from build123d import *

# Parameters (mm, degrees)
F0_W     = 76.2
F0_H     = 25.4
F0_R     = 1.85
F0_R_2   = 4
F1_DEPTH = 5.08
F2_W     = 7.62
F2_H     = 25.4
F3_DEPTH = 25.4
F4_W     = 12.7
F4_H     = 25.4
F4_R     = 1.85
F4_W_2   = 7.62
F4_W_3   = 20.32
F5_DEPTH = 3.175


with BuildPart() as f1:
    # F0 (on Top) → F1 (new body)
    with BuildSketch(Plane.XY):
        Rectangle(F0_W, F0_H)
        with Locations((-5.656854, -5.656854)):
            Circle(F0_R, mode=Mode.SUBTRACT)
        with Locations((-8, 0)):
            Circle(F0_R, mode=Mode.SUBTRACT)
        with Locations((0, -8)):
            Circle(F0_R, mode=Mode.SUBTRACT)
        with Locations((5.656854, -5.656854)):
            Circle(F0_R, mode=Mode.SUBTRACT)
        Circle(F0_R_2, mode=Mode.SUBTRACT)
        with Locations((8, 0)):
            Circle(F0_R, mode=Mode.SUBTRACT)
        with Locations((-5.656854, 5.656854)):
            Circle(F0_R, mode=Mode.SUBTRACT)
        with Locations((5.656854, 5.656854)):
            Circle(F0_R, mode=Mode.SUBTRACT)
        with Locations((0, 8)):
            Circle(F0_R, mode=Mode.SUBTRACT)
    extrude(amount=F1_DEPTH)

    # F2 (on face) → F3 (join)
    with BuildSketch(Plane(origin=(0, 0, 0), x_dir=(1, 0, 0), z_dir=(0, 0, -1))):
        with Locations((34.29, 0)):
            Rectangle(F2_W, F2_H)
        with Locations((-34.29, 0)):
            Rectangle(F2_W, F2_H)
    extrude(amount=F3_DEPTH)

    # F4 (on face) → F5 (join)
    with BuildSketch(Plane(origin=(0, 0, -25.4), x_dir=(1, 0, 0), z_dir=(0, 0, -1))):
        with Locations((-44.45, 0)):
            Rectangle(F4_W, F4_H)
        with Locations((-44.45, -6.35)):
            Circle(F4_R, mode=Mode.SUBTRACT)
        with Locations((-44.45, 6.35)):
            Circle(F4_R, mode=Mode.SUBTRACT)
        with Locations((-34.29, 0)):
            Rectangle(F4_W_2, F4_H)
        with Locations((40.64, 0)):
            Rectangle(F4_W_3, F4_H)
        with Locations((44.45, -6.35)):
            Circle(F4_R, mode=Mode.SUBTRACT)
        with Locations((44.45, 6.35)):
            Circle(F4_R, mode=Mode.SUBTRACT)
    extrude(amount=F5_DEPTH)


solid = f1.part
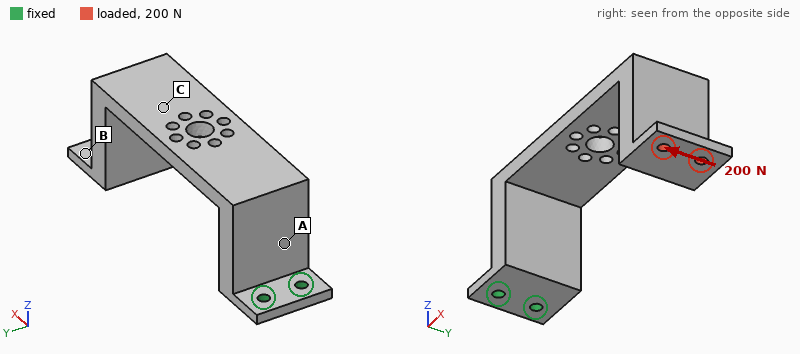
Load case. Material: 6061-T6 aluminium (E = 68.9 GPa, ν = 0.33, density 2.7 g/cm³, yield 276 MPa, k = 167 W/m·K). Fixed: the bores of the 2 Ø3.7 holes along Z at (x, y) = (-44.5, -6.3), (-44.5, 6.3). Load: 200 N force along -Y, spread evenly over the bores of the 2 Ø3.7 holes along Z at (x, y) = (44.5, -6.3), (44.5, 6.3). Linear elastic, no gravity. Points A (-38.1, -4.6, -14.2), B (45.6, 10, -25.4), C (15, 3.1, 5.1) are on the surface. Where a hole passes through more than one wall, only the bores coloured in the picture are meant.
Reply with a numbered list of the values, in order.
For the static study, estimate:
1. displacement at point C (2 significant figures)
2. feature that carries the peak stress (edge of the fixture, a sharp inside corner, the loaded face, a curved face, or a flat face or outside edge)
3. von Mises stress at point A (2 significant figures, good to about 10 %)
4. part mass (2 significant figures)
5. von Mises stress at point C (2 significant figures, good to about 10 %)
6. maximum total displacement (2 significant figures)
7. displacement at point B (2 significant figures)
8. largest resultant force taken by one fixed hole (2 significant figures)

1. 0.30 mm
2. a curved face
3. 64 MPa
4. 60 g
5. 55 MPa
6. 1.2 mm
7. 1.1 mm
8. 1.2 kN
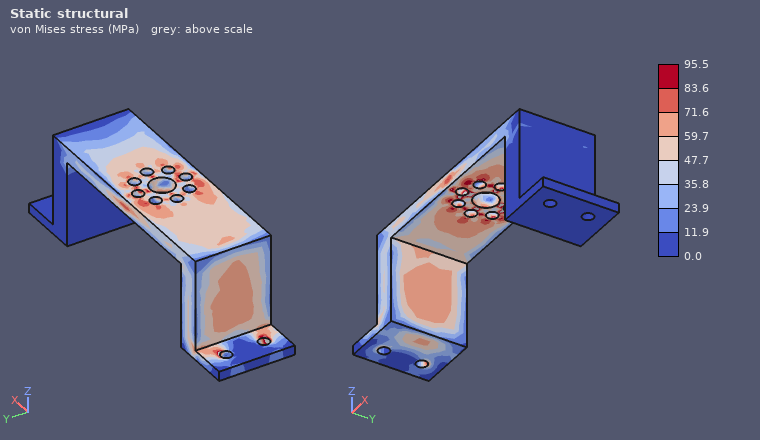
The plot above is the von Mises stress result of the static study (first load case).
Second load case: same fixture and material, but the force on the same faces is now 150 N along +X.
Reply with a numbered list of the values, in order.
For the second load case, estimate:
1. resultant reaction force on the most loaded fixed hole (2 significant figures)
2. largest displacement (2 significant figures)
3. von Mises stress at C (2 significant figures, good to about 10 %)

1. 75 N
2. 1.2 mm
3. 37 MPa
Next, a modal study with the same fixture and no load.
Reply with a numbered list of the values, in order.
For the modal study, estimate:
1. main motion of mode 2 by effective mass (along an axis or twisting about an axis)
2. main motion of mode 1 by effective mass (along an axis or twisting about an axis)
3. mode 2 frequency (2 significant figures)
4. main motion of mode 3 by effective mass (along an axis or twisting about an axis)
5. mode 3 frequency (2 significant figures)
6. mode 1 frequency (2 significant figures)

1. along Y
2. along Z
3. 580 Hz
4. along X
5. 740 Hz
6. 230 Hz
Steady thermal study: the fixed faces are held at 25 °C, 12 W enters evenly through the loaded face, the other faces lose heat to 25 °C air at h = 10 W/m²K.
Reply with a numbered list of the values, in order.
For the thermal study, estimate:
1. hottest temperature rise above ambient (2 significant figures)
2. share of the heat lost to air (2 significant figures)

1. 66 K
2. 26 %
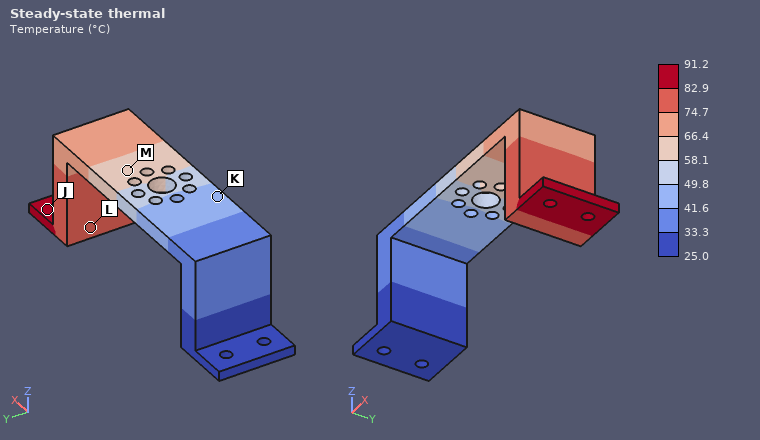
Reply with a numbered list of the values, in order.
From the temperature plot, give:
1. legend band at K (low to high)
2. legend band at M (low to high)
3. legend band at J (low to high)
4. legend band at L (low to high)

1. 41.6 to 49.8 °C
2. 58.1 to 66.4 °C
3. 82.9 to 91.2 °C
4. 74.7 to 82.9 °C
